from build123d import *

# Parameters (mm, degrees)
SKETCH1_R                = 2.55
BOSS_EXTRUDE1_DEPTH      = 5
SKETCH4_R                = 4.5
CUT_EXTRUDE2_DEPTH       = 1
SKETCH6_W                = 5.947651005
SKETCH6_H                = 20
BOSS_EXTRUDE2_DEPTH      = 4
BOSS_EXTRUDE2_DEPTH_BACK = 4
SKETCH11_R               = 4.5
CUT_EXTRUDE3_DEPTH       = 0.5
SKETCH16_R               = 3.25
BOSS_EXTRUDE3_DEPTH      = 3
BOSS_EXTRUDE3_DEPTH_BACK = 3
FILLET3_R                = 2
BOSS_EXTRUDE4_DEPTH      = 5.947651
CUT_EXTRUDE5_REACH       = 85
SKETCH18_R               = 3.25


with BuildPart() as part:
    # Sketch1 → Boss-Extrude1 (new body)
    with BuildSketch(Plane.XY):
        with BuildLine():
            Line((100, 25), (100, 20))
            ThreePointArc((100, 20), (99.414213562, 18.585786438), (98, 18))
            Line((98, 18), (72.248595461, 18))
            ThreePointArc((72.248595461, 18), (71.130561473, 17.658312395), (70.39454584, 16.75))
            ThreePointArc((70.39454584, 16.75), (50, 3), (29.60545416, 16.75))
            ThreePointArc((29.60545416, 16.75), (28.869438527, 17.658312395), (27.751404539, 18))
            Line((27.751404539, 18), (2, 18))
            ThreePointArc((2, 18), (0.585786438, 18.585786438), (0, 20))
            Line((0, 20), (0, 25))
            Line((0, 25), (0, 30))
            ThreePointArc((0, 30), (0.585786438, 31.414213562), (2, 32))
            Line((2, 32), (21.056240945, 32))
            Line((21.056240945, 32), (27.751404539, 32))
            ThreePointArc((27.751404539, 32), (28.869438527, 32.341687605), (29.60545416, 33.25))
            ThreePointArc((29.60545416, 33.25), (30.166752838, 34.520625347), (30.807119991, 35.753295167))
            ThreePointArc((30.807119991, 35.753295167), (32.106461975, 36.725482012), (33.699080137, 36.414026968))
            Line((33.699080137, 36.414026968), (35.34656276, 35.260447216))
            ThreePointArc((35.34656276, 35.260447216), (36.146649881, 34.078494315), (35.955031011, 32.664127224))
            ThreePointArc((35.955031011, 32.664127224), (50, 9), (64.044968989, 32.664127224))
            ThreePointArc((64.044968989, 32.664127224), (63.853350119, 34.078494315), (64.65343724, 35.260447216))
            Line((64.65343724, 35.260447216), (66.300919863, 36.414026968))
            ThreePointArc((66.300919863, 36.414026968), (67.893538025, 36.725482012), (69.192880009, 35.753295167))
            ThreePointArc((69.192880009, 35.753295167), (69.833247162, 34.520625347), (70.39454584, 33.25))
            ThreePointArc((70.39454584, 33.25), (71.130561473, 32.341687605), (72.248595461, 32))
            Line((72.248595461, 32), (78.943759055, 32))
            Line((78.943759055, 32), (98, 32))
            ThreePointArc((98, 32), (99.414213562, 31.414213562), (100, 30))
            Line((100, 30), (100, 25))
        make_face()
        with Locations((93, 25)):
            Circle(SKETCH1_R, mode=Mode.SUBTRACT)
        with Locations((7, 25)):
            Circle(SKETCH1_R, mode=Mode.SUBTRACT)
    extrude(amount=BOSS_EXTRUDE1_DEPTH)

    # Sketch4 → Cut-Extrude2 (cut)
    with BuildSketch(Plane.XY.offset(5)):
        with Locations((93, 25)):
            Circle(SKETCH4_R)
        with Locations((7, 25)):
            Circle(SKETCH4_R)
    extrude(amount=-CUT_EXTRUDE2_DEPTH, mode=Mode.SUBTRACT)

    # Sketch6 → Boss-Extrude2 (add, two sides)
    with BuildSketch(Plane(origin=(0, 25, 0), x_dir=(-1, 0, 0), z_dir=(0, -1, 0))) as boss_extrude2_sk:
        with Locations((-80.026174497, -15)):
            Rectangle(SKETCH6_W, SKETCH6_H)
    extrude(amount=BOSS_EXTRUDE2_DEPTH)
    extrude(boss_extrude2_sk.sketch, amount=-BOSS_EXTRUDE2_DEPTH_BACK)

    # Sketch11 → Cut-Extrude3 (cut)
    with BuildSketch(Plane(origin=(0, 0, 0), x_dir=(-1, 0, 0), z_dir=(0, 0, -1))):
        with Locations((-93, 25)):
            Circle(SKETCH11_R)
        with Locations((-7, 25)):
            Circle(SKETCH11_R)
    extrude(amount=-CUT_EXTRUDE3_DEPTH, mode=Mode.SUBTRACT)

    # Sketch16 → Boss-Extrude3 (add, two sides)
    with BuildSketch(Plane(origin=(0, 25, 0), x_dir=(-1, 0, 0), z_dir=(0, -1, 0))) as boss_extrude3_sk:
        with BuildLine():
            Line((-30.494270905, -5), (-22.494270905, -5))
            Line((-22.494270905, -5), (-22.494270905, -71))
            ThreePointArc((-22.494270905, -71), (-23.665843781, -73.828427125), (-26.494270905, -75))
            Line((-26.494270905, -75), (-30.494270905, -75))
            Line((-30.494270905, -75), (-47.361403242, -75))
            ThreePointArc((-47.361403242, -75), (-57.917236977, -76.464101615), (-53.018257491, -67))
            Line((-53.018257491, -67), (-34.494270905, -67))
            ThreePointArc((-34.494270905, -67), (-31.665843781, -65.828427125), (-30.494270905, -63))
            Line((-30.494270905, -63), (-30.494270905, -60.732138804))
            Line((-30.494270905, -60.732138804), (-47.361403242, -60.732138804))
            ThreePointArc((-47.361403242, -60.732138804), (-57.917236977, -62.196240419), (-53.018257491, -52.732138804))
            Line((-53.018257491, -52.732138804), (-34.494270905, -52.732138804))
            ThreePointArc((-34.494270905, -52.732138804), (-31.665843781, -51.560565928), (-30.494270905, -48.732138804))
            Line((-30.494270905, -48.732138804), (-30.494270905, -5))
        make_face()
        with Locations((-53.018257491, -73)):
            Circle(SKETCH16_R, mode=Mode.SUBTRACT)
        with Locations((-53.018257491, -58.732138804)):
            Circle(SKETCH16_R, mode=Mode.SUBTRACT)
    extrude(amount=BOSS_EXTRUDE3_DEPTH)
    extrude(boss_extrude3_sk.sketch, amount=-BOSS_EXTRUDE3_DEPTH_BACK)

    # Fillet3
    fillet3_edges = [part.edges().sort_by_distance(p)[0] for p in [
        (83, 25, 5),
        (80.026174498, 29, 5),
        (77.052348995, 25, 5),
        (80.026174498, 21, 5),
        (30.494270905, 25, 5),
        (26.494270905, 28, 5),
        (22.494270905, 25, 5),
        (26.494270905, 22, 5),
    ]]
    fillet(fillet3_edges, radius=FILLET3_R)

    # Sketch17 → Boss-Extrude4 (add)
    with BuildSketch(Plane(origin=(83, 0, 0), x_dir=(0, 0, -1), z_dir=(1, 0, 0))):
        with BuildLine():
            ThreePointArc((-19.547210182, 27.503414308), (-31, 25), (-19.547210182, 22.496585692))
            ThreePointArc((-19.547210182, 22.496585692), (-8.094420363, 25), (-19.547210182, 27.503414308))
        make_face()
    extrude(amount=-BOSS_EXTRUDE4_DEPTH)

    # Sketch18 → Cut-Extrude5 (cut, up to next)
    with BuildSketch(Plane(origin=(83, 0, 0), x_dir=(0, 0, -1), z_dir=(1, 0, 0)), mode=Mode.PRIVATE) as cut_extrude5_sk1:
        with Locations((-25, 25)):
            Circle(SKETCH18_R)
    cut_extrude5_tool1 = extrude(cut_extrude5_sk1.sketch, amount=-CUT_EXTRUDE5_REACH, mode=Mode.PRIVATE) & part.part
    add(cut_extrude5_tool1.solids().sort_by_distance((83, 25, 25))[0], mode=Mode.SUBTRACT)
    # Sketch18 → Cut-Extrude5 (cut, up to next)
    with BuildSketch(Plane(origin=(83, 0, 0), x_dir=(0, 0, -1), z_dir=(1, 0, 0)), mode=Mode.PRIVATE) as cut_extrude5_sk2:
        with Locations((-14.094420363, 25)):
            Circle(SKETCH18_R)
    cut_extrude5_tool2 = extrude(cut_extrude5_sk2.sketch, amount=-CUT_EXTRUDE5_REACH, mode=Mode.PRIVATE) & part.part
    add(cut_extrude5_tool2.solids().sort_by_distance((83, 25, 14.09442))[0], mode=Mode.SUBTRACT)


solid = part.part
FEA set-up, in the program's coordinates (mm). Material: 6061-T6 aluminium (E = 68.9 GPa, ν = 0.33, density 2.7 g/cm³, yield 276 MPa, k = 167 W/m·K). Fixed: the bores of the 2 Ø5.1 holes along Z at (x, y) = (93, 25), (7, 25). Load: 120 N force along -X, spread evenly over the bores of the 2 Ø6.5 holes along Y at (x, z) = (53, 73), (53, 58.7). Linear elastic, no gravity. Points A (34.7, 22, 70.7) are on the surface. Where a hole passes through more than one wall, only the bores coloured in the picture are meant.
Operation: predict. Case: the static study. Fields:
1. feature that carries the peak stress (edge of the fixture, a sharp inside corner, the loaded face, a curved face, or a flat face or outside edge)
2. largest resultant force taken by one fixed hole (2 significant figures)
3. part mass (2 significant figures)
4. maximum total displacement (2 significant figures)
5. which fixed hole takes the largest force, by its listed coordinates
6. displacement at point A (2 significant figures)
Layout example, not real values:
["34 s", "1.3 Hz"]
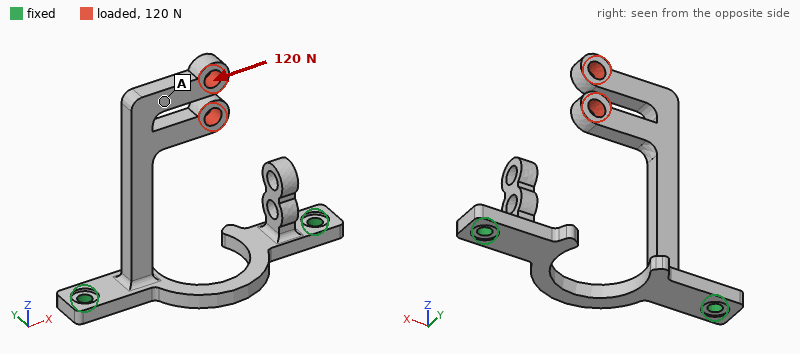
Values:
["a curved face", "130 N", "36 g", "1.5 mm", "(7, 25)", "1.2 mm"]
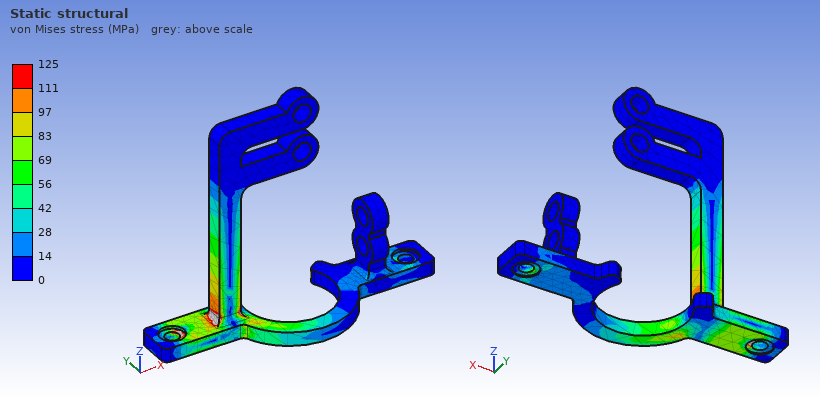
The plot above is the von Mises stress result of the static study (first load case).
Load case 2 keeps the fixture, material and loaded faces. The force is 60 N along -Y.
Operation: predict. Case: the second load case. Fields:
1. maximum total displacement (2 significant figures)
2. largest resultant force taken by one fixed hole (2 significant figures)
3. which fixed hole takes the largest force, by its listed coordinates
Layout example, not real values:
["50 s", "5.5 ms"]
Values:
["1.3 mm", "55 N", "(7, 25)"]
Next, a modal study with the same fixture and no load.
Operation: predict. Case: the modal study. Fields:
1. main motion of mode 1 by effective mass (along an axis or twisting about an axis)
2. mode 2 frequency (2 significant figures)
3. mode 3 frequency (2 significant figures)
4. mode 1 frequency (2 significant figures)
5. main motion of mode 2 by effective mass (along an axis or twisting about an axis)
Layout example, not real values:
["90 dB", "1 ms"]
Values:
["along Y", "480 Hz", "1800 Hz", "410 Hz", "along X"]
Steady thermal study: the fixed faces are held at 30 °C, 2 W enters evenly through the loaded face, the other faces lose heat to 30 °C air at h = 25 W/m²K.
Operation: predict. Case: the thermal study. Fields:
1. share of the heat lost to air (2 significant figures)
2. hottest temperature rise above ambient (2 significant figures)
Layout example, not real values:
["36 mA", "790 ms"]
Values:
["43 %", "13 K"]
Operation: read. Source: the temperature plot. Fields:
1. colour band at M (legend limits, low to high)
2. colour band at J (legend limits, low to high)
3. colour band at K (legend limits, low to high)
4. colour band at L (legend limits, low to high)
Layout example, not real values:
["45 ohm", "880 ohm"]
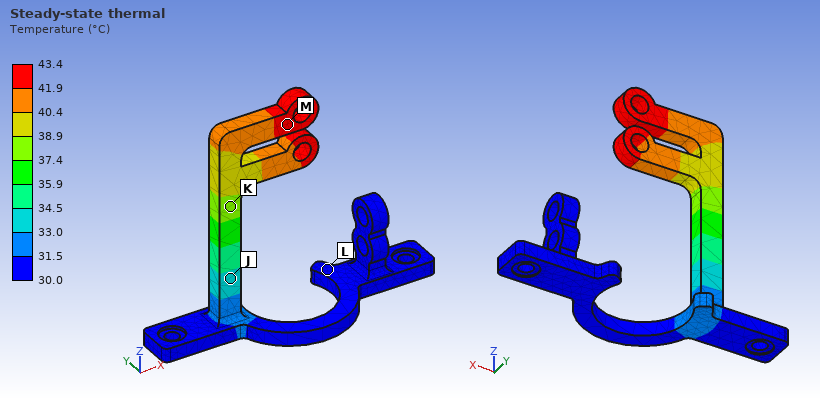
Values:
["41.9 to 43.4 °C", "33.0 to 34.5 °C", "37.4 to 38.9 °C", "30.0 to 31.5 °C"]
